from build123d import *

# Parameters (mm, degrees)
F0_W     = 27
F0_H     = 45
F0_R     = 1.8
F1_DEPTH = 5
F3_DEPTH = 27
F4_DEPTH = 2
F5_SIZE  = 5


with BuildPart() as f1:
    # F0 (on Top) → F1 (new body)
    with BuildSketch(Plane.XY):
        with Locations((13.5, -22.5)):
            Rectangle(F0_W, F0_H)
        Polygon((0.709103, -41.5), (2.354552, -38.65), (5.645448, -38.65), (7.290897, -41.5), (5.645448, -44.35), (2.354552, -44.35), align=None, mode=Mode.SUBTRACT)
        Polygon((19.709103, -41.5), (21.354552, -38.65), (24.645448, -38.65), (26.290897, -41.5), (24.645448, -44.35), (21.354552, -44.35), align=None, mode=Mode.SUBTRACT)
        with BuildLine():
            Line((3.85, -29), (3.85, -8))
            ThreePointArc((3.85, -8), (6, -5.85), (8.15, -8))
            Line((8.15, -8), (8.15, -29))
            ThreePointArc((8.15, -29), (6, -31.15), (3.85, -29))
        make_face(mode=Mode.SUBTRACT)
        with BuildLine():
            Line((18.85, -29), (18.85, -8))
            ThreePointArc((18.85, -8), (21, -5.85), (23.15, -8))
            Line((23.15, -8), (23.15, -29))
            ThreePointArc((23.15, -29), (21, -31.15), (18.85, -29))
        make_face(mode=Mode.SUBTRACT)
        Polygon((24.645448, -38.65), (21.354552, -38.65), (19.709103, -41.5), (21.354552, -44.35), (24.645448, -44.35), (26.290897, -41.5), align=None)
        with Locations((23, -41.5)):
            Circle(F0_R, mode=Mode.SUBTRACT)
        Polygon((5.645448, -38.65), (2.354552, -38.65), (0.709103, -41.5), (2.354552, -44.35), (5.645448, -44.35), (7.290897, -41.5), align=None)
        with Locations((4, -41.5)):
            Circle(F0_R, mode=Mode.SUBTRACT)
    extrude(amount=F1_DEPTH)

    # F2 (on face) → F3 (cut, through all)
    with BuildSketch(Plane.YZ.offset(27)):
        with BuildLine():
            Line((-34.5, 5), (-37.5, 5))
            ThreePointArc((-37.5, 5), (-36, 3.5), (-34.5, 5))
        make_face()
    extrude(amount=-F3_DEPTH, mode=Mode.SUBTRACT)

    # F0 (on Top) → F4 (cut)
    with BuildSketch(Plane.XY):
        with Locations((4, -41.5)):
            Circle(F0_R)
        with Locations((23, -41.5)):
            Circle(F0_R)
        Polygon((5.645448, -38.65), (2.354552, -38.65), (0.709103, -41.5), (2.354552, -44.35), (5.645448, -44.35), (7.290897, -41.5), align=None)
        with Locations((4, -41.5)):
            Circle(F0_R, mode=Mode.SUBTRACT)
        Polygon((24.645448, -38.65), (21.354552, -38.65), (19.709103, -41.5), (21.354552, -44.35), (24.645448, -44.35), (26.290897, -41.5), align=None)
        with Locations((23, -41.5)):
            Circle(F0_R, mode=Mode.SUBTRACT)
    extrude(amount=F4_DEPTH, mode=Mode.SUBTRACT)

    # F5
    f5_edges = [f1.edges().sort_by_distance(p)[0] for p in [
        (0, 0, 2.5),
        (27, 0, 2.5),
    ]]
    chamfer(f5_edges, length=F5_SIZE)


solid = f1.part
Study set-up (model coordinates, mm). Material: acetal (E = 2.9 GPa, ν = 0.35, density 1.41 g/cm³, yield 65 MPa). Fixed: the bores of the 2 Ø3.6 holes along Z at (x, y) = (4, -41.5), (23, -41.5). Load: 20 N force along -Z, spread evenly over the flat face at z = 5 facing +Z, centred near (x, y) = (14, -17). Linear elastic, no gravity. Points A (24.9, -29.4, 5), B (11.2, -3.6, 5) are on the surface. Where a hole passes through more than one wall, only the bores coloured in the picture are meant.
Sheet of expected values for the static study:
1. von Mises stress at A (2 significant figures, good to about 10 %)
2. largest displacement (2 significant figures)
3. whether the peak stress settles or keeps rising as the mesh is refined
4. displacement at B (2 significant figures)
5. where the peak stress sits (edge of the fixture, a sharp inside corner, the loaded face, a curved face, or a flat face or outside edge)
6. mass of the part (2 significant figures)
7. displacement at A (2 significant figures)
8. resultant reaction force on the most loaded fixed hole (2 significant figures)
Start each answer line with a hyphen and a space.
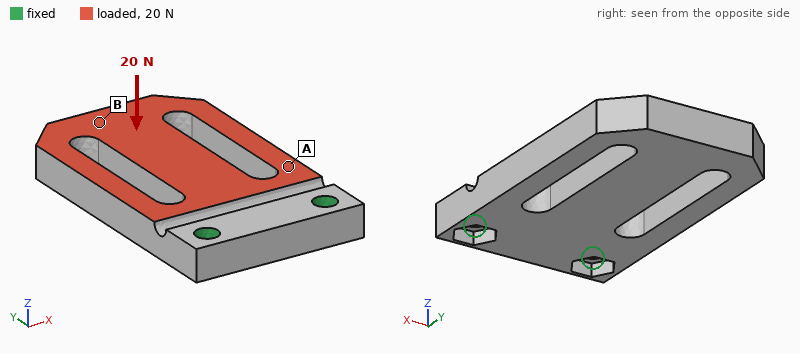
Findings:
- 3.1 MPa
- 0.57 mm
- keeps rising
- 0.50 mm
- edge of the fixture
- 6.5 g
- 0.098 mm
- 10 N
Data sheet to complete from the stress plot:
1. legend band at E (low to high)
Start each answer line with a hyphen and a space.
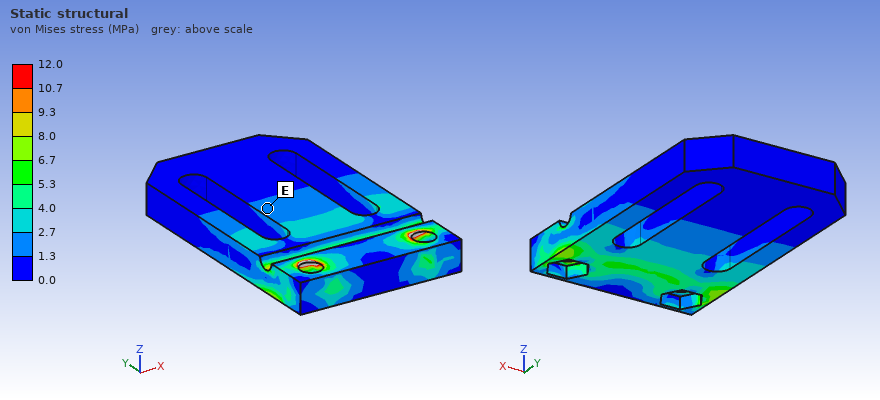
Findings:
- 1.3 to 2.7 MPa
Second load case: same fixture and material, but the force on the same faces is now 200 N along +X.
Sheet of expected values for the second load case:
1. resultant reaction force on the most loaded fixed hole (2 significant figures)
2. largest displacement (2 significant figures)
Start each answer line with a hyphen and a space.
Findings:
- 250 N
- 0.45 mm
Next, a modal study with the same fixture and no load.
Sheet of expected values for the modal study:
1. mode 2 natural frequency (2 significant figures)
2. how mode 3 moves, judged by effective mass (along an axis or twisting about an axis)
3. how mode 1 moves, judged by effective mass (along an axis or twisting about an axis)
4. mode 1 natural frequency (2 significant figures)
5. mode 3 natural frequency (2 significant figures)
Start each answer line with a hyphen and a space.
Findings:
- 1800 Hz
- along X
- along Z
- 520 Hz
- 2000 Hz
